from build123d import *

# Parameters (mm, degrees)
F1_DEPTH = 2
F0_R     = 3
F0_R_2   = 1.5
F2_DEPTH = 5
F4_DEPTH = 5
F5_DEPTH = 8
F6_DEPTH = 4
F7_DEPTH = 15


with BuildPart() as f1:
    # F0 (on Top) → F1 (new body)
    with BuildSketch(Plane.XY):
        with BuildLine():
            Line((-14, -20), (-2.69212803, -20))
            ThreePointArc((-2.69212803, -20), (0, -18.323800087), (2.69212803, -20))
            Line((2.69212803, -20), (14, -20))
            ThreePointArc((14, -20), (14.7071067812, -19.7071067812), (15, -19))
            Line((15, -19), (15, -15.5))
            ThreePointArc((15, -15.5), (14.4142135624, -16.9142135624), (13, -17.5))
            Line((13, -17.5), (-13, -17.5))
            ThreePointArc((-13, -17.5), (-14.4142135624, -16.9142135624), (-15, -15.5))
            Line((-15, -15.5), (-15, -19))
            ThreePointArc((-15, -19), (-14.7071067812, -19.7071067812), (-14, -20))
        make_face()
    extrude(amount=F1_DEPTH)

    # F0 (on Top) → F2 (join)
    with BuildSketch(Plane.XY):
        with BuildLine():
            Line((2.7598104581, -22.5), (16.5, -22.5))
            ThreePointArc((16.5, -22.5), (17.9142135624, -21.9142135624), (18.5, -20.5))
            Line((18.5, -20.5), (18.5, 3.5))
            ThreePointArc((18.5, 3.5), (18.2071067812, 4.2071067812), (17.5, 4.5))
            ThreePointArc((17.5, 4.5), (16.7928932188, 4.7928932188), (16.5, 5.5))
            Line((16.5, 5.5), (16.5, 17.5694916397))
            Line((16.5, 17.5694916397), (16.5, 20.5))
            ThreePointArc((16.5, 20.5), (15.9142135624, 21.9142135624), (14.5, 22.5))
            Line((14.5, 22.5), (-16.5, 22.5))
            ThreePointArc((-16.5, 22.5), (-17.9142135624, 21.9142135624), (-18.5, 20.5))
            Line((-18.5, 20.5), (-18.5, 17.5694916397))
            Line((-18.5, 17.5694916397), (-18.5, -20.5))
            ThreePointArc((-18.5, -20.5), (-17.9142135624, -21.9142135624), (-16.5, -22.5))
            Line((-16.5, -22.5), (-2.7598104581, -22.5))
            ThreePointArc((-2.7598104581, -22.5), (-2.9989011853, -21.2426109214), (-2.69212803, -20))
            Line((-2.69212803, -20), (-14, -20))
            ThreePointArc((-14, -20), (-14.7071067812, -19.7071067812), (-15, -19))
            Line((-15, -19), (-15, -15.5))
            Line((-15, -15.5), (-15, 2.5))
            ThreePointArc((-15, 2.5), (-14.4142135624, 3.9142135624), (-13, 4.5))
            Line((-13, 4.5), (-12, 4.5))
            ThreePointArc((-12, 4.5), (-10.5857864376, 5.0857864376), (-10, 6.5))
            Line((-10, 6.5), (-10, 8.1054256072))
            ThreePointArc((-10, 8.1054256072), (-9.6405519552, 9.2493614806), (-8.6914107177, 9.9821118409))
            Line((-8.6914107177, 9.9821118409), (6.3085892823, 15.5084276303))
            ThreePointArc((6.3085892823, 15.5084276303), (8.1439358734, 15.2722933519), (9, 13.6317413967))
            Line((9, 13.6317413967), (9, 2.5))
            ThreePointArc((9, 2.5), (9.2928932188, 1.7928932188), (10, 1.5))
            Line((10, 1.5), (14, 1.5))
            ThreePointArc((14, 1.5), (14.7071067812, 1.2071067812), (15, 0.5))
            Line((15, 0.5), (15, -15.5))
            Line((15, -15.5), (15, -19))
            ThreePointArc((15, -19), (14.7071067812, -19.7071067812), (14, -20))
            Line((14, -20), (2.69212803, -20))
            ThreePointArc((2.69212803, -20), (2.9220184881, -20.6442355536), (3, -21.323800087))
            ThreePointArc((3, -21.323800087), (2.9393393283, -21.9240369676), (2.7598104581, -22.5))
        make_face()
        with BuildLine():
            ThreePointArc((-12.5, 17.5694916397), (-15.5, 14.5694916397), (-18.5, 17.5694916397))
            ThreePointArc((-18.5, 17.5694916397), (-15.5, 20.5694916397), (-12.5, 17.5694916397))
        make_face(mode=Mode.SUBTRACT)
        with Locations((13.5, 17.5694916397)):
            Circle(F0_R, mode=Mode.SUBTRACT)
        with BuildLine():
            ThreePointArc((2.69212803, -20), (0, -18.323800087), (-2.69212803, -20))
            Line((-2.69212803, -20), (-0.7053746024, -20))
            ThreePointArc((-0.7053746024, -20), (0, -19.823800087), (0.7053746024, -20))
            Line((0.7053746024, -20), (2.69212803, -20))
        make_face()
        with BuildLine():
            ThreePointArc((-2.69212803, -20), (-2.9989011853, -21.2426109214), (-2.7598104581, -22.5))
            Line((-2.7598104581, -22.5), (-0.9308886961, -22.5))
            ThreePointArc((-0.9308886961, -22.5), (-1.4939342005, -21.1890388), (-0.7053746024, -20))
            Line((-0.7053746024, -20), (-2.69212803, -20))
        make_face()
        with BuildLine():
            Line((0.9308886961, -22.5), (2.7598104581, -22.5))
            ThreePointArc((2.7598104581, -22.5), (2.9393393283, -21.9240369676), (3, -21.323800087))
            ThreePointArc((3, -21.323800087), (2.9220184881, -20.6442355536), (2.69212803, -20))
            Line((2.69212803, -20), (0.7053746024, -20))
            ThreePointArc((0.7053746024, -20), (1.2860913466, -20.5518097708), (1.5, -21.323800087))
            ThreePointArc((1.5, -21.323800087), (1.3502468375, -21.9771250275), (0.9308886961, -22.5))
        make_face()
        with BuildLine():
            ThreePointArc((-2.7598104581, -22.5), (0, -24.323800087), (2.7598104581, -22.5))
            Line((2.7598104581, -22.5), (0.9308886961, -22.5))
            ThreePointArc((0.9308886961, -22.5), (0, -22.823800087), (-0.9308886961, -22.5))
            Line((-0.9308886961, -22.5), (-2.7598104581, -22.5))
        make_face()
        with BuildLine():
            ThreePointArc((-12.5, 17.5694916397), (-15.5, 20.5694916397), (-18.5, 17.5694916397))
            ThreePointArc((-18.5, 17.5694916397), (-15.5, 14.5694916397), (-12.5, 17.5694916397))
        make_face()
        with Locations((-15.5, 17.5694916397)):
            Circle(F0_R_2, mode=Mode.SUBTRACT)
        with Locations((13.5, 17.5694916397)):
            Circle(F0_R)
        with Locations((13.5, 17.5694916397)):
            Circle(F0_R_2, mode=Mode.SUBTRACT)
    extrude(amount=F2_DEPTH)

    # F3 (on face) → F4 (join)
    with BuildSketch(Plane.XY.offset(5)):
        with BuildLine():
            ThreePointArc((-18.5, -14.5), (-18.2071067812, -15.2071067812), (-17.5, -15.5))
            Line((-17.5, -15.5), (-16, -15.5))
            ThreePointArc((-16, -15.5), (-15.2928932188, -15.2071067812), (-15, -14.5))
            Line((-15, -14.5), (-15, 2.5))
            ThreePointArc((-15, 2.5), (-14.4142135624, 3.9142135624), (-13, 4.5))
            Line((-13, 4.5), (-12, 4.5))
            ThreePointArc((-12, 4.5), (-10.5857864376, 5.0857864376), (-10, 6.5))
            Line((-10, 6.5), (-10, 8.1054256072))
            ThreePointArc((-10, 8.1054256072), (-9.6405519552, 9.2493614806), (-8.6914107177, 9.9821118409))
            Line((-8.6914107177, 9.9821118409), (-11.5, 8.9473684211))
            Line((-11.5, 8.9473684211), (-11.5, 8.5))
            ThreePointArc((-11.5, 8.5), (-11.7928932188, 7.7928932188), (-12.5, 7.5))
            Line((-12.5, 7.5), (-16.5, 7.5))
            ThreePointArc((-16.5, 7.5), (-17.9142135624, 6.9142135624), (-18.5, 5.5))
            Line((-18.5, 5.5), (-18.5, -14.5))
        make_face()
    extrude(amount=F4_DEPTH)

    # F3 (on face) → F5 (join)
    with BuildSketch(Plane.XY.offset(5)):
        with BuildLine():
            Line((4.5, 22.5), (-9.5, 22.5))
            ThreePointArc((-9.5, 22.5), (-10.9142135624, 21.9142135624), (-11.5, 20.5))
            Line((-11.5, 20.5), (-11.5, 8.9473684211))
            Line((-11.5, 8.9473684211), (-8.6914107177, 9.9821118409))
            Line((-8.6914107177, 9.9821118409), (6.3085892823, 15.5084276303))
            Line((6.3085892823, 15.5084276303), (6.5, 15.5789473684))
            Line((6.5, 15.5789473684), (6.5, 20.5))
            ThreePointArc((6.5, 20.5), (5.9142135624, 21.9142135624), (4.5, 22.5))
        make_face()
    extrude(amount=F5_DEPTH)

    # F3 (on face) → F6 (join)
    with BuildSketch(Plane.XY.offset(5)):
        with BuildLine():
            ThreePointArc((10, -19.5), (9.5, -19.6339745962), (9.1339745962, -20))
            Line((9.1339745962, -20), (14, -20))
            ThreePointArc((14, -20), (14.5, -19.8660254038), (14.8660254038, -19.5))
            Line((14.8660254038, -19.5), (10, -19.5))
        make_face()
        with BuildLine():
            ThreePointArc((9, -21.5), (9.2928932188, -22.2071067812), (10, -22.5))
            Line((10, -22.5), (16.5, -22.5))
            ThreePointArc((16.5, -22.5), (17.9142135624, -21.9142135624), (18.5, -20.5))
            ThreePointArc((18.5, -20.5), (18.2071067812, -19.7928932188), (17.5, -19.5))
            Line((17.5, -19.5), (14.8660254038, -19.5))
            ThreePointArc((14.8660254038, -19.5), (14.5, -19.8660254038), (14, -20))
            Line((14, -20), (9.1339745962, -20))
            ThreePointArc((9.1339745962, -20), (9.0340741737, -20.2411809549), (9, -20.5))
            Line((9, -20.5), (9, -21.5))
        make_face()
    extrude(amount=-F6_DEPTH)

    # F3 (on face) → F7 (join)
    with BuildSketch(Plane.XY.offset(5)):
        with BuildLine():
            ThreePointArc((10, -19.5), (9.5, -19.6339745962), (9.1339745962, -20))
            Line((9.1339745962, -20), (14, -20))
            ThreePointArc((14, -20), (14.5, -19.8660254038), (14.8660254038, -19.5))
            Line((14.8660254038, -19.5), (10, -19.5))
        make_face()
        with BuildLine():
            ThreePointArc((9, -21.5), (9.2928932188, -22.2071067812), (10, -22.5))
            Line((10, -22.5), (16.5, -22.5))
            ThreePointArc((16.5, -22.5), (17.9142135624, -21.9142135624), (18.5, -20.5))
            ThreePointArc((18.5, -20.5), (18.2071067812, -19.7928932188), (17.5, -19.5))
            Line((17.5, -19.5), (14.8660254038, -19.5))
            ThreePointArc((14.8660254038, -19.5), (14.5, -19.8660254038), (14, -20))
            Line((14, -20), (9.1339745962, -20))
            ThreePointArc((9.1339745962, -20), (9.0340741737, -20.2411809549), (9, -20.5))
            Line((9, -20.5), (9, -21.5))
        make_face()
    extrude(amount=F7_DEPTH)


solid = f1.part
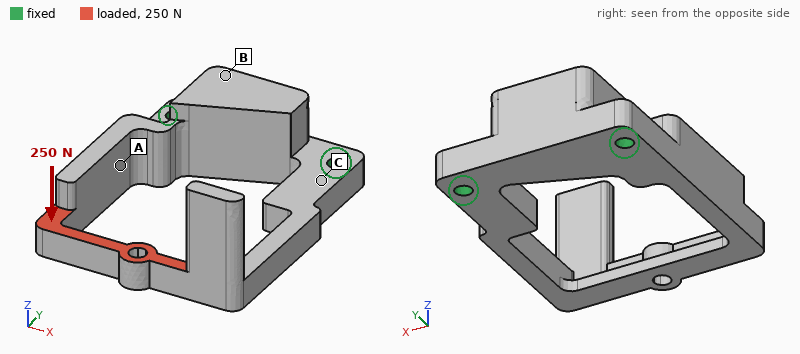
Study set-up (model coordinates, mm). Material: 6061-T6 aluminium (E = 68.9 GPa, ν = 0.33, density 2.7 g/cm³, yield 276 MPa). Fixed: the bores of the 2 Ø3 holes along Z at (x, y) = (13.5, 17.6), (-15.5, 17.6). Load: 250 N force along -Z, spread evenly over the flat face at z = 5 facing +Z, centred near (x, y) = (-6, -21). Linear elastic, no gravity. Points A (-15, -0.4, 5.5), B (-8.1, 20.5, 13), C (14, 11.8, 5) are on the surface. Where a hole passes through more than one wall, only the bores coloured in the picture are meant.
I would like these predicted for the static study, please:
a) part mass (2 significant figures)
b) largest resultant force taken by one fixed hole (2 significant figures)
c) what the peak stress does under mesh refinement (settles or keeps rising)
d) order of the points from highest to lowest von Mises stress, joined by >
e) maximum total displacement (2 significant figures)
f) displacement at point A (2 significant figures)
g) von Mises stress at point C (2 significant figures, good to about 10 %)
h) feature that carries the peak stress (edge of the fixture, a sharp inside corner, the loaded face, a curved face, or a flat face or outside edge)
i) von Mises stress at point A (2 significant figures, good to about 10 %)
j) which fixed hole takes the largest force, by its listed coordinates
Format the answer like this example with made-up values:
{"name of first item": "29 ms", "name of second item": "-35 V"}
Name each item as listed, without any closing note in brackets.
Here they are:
{"part mass": "17 g", "largest resultant force taken by one fixed hole": "200 N", "what the peak stress does under mesh refinement": "keeps rising", "order of the points from highest to lowest von Mises stress, joined by >": "C > A > B", "maximum total displacement": "0.46 mm", "displacement at point A": "0.091 mm", "von Mises stress at point C": "76 MPa", "feature that carries the peak stress": "a sharp inside corner", "von Mises stress at point A": "40 MPa", "which fixed hole takes the largest force, by its listed coordinates": "(-15.5, 17.6)"}
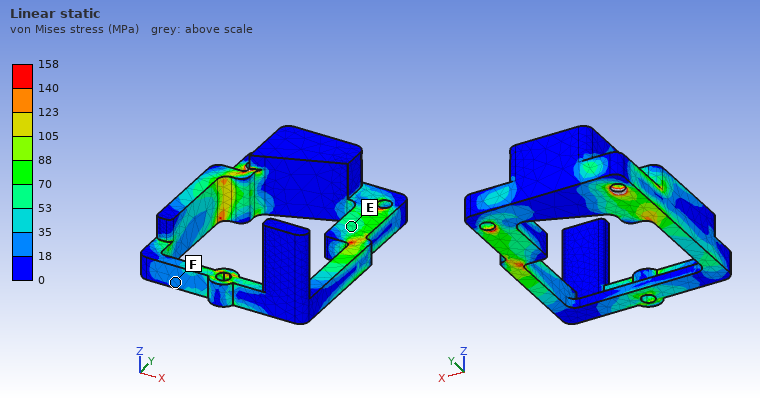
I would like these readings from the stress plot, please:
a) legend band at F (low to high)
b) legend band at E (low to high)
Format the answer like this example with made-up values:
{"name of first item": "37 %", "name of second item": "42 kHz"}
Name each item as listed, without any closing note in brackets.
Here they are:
{"legend band at F": "18 to 35 MPa", "legend band at E": "53 to 70 MPa"}
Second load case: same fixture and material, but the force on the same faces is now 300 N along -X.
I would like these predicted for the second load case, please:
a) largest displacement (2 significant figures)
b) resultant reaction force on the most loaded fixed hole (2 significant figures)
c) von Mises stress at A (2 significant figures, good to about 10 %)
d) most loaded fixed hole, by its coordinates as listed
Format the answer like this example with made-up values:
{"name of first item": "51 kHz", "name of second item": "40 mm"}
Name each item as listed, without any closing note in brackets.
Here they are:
{"largest displacement": "0.26 mm", "resultant reaction force on the most loaded fixed hole": "380 N", "von Mises stress at A": "79 MPa", "most loaded fixed hole, by its coordinates as listed": "(13.5, 17.6)"}
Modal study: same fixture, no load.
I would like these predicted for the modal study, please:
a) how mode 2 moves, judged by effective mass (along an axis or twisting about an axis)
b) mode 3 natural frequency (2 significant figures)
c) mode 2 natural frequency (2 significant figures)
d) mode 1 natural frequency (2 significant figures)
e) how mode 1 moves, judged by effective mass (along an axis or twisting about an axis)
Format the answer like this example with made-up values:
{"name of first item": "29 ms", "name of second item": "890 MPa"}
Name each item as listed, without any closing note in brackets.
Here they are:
{"how mode 2 moves, judged by effective mass": "along X", "mode 3 natural frequency": "3900 Hz", "mode 2 natural frequency": "2900 Hz", "mode 1 natural frequency": "1800 Hz", "how mode 1 moves, judged by effective mass": "along Z"}
